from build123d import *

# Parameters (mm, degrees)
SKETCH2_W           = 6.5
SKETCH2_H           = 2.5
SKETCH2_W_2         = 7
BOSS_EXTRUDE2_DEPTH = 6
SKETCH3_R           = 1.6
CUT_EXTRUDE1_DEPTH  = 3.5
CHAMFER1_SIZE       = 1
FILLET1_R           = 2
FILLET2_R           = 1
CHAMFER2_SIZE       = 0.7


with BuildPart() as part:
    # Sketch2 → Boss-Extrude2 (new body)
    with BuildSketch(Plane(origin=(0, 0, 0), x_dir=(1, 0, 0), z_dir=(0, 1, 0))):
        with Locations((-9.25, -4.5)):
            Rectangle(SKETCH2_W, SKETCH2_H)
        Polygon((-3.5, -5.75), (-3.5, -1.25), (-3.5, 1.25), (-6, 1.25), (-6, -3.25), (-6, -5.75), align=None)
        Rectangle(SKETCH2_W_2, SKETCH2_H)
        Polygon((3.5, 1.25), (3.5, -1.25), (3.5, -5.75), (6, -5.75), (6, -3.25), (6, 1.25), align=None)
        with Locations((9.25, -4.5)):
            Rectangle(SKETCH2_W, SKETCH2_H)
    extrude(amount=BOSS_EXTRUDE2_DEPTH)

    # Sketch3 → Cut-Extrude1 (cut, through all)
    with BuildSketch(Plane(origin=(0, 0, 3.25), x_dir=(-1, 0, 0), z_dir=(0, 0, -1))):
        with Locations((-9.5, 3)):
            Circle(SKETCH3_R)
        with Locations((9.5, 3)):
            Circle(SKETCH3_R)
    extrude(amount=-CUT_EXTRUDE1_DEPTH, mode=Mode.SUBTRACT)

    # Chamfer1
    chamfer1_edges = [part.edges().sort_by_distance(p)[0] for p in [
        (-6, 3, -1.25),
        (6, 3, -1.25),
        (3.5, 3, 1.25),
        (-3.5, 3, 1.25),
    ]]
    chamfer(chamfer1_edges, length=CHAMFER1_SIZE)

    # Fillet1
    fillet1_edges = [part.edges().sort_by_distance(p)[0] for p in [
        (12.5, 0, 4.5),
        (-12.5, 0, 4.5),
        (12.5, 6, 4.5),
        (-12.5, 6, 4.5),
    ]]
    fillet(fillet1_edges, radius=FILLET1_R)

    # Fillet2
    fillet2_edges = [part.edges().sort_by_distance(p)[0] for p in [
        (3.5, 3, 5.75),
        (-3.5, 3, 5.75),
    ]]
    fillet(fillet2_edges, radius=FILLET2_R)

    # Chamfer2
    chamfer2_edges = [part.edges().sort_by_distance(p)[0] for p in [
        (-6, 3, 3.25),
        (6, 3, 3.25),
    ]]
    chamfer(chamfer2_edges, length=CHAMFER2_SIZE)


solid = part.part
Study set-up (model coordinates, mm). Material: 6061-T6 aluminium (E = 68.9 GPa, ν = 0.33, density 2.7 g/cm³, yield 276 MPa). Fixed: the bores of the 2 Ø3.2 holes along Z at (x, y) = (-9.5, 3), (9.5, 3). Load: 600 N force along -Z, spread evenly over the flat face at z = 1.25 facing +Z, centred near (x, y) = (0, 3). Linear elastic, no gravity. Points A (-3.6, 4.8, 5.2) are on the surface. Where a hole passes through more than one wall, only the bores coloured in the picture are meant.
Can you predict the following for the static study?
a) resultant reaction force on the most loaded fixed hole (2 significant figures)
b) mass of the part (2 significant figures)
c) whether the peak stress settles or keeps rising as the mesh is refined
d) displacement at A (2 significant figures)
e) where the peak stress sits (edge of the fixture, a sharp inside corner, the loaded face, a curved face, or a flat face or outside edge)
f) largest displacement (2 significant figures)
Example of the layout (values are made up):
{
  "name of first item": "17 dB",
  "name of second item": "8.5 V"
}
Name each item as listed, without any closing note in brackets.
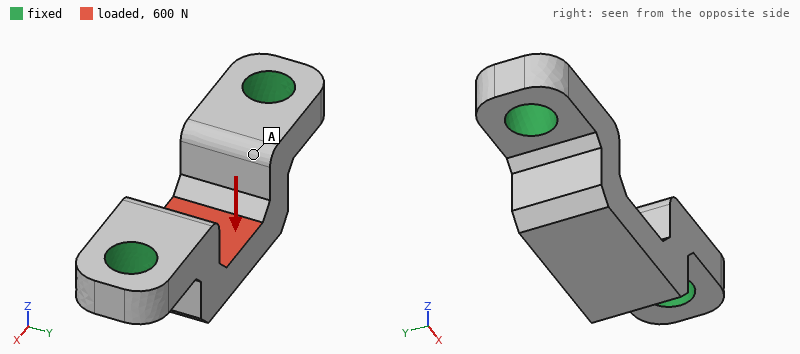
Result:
{
  "resultant reaction force on the most loaded fixed hole": "420 N",
  "mass of the part": "1.2 g",
  "whether the peak stress settles or keeps rising as the mesh is refined": "keeps rising",
  "displacement at A": "5.5 µm",
  "where the peak stress sits": "edge of the fixture",
  "largest displacement": "11 µm"
}
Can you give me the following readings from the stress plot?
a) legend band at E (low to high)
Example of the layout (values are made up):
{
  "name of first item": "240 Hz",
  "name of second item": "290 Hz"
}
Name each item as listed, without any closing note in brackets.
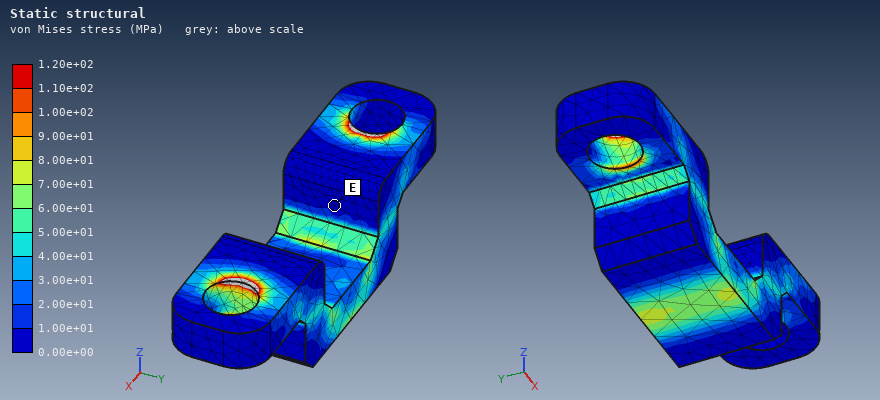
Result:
{
  "legend band at E": "0.00e+00 to 1.00e+01 MPa"
}
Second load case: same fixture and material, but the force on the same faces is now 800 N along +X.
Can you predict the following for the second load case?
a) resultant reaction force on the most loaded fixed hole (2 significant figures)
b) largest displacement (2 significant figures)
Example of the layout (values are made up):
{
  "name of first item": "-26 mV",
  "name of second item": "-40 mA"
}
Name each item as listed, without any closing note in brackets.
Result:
{
  "resultant reaction force on the most loaded fixed hole": "420 N",
  "largest displacement": "14 µm"
}
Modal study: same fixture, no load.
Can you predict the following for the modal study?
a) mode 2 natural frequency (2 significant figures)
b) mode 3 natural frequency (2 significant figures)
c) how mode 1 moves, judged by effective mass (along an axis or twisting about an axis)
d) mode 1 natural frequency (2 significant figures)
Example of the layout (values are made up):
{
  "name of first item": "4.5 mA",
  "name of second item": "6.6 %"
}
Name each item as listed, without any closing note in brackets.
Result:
{
  "mode 2 natural frequency": "56 kHz",
  "mode 3 natural frequency": "57 kHz",
  "how mode 1 moves, judged by effective mass": "along Y",
  "mode 1 natural frequency": "28 kHz"
}
